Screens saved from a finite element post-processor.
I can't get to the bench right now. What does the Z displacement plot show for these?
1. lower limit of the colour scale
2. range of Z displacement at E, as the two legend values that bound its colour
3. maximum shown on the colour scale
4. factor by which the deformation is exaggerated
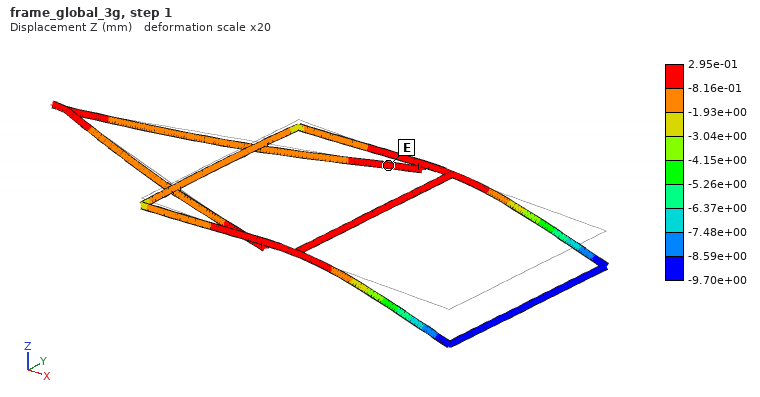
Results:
-9.70e+00 mm
-8.16e-01 to 2.95e-01 mm
2.95e-01 mm
20
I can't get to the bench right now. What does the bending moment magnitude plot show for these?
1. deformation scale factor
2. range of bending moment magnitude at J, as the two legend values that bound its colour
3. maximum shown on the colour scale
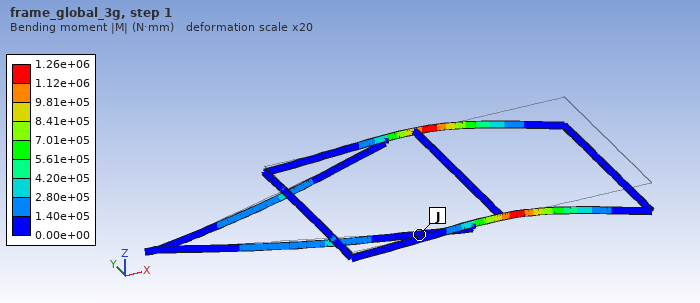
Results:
20
0.00e+00 to 1.40e+05 N·mm
1.26e+06 N·mm
